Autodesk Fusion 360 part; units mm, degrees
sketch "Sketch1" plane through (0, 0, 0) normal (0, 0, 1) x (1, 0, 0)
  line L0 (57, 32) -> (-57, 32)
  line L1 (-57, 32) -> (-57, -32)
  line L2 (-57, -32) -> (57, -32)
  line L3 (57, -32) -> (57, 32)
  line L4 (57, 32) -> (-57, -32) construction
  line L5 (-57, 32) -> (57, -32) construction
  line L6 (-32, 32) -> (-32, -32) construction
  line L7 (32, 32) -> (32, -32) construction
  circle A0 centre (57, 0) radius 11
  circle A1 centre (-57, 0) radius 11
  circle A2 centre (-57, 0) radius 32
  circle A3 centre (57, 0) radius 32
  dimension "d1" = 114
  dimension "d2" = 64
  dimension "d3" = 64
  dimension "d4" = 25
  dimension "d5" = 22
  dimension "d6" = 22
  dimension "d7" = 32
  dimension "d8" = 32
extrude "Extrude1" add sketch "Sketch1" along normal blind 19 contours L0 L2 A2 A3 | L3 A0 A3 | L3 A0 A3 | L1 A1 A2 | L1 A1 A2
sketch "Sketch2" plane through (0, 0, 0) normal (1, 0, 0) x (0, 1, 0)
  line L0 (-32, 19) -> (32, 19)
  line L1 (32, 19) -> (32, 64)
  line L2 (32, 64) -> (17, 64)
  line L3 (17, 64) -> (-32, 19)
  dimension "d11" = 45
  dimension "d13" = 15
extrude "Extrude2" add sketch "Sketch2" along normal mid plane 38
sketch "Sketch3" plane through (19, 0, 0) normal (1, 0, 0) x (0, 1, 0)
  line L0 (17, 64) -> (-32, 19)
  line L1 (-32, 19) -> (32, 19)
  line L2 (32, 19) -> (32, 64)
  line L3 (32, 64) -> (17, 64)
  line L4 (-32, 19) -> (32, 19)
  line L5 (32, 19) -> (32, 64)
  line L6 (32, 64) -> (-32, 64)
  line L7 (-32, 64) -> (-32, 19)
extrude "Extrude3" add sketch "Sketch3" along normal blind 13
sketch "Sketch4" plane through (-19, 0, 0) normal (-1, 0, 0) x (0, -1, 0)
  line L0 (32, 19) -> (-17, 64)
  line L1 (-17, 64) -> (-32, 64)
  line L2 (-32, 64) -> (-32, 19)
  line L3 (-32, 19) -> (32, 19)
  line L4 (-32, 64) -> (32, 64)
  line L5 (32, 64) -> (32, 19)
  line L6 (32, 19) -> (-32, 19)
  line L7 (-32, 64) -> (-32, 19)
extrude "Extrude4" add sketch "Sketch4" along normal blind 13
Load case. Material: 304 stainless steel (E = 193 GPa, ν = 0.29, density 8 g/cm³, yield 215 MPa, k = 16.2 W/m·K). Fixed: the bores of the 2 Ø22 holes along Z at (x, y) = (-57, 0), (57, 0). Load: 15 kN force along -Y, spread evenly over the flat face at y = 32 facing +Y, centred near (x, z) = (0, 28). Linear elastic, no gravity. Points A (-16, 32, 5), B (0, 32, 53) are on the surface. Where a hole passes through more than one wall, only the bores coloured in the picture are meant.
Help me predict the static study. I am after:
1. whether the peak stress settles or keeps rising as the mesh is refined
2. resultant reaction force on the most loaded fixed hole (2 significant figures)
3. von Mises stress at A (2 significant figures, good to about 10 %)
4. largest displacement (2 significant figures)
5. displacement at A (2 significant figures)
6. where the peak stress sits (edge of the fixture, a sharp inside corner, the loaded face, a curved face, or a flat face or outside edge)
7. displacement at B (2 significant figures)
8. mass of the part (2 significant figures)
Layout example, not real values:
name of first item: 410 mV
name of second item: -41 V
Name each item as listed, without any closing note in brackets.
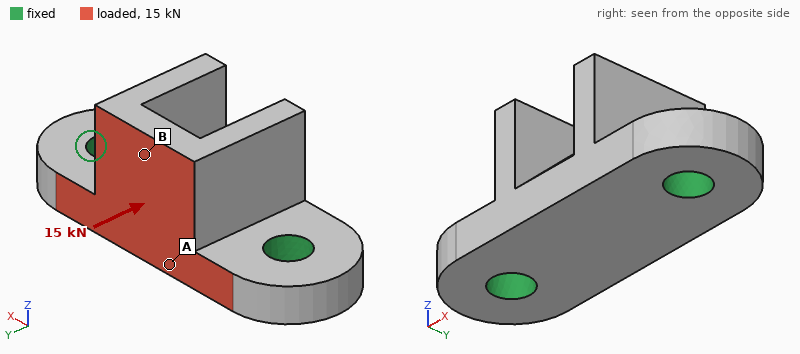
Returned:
whether the peak stress settles or keeps rising as the mesh is refined: keeps rising
resultant reaction force on the most loaded fixed hole: 7.5 kN
von Mises stress at A: 12 MPa
largest displacement: 23 µm
displacement at A: 9.5 µm
where the peak stress sits: edge of the fixture
displacement at B: 20 µm
mass of the part: 2.6 kg
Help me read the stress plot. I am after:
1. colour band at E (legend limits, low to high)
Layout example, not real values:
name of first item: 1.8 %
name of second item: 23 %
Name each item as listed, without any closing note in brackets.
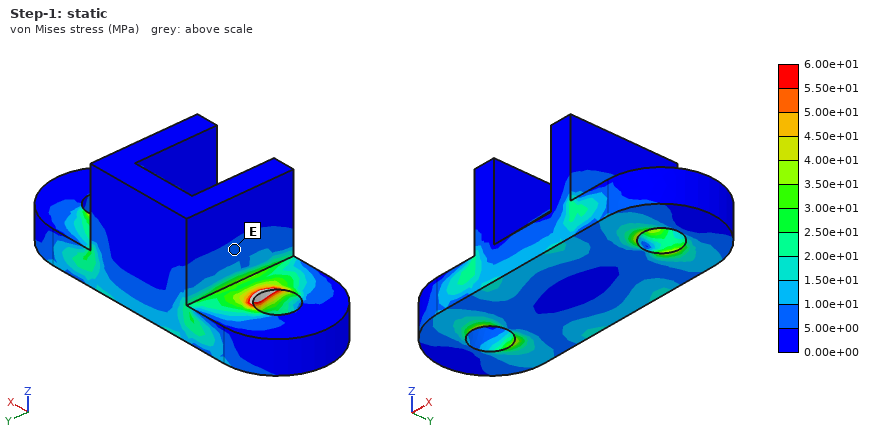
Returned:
colour band at E: 5.00e+00 to 1.00e+01 MPa
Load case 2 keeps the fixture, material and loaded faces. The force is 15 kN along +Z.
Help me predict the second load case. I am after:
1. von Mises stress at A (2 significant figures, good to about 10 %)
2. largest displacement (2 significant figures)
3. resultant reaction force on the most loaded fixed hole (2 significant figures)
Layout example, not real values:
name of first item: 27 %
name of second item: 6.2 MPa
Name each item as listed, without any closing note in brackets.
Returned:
von Mises stress at A: 9.9 MPa
largest displacement: 34 µm
resultant reaction force on the most loaded fixed hole: 7.9 kN
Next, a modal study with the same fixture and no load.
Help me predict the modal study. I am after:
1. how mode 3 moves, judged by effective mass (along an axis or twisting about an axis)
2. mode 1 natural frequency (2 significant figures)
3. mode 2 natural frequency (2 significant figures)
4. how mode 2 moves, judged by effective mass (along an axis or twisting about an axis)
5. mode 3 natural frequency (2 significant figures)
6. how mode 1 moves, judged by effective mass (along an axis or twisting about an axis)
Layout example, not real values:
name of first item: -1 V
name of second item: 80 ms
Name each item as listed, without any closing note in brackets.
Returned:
how mode 3 moves, judged by effective mass: along X
mode 1 natural frequency: 3400 Hz
mode 2 natural frequency: 6100 Hz
how mode 2 moves, judged by effective mass: along Z
mode 3 natural frequency: 6900 Hz
how mode 1 moves, judged by effective mass: along Y
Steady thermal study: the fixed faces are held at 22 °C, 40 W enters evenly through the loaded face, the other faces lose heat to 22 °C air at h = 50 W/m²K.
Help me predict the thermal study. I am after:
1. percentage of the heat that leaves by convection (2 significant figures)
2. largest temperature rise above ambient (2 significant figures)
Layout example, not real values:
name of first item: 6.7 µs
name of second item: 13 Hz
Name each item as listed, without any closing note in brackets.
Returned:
percentage of the heat that leaves by convection: 45 %
largest temperature rise above ambient: 31 K
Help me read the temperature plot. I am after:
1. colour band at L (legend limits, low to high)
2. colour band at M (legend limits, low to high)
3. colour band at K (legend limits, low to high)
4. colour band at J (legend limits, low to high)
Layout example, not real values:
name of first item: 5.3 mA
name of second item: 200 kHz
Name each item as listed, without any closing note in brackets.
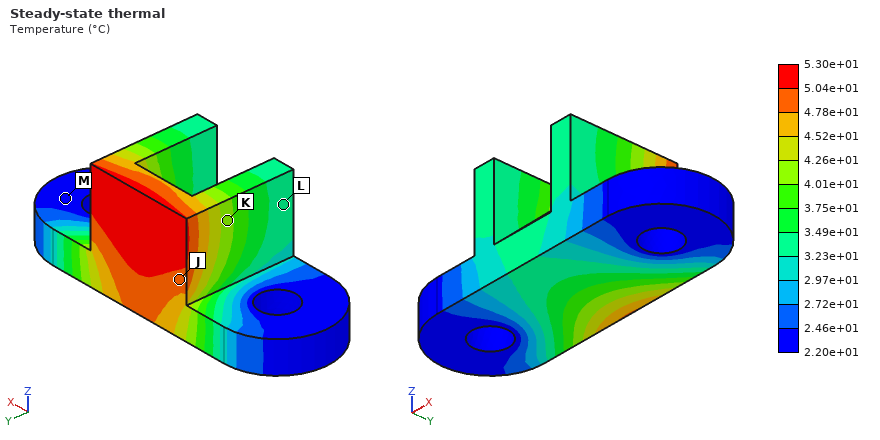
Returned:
colour band at L: 3.23e+01 to 3.49e+01 °C
colour band at M: 2.20e+01 to 2.46e+01 °C
colour band at K: 4.01e+01 to 4.26e+01 °C
colour band at J: 4.78e+01 to 5.04e+01 °C
